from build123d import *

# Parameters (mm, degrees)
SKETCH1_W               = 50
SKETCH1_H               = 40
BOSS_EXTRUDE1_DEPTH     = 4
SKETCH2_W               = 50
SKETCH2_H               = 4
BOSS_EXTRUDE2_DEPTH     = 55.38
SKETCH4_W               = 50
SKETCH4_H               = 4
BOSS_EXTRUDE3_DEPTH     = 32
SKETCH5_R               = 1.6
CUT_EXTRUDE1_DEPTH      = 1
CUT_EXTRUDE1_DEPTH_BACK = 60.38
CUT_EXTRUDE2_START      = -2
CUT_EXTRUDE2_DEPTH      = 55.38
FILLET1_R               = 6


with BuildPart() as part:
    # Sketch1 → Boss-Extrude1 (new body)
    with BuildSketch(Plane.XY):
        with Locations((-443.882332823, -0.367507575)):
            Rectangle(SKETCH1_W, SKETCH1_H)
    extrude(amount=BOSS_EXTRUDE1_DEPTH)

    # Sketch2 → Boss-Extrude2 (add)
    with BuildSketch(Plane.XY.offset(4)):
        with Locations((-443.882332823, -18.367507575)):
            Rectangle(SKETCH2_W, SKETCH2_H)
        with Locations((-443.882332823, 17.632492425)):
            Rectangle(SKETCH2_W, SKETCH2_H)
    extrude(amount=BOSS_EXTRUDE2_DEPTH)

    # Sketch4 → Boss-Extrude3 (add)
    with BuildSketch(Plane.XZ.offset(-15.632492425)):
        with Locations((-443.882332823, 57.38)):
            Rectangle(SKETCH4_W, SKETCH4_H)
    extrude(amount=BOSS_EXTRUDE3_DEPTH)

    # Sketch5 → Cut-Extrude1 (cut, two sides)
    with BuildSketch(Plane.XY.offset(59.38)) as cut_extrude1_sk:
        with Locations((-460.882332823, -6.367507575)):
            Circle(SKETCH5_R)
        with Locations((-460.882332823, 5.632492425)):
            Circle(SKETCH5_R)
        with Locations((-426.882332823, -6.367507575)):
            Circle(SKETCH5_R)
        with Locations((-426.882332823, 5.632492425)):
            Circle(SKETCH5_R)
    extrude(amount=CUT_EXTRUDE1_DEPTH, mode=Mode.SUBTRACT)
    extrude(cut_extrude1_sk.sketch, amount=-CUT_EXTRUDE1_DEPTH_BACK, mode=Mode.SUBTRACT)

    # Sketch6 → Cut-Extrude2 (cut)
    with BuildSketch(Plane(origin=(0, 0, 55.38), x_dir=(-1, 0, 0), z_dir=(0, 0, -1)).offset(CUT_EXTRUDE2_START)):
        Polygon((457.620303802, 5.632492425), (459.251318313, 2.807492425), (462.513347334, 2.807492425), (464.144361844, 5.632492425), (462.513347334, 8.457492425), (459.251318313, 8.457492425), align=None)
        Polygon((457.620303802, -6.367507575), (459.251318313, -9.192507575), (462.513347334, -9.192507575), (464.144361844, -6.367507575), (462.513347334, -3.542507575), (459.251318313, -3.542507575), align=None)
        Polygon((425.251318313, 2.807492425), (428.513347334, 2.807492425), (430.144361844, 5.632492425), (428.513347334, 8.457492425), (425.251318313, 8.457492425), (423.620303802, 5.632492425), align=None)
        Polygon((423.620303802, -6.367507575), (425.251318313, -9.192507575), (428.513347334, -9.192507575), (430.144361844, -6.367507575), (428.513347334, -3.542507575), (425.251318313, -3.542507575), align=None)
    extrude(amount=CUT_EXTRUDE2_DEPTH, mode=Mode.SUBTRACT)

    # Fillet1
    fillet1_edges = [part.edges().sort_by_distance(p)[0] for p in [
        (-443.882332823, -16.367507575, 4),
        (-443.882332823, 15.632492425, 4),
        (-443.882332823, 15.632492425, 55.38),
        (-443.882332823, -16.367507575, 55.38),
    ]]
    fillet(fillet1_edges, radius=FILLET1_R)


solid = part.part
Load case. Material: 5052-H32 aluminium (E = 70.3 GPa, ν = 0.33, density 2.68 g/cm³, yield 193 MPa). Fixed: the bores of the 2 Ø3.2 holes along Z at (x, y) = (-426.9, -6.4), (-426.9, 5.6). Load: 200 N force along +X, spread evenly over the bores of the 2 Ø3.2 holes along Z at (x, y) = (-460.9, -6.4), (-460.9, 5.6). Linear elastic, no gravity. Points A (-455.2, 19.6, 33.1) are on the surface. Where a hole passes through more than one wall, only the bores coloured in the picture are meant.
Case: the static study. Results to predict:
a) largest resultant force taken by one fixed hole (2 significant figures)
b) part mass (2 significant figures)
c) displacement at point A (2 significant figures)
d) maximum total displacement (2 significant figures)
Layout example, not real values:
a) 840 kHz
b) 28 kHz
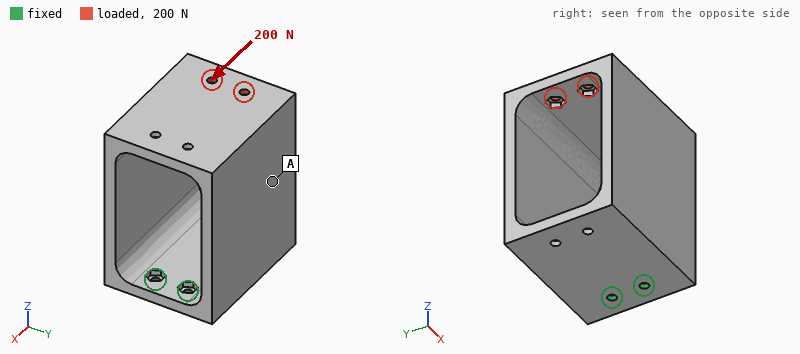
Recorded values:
a) 180 N
b) 100 g
c) 0.39 mm
d) 0.67 mm
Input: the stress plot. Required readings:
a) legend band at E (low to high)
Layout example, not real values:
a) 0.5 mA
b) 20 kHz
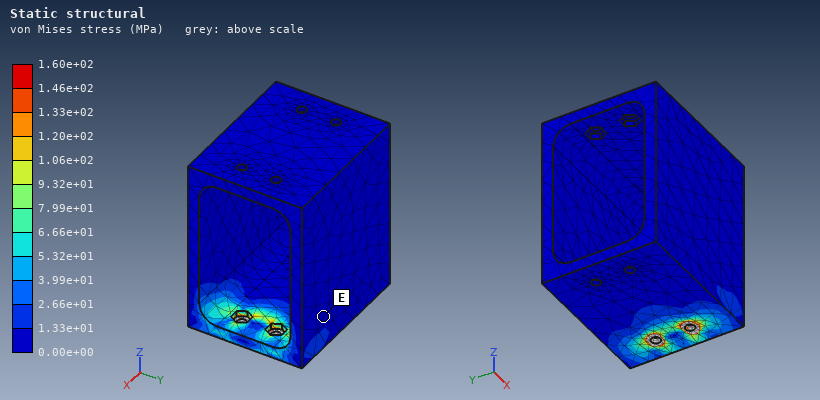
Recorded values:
a) 0.00e+00 to 1.33e+01 MPa
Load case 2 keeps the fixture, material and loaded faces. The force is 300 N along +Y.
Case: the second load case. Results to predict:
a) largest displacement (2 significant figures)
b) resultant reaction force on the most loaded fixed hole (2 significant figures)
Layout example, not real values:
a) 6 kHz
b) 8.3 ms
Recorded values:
a) 0.39 mm
b) 1.3 kN
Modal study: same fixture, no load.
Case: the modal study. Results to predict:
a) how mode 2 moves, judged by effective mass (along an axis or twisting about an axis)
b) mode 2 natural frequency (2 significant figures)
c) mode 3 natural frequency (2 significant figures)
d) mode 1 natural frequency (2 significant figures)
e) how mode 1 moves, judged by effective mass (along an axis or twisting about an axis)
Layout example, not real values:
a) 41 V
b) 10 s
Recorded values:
a) along Y
b) 650 Hz
c) 2000 Hz
d) 420 Hz
e) along X
